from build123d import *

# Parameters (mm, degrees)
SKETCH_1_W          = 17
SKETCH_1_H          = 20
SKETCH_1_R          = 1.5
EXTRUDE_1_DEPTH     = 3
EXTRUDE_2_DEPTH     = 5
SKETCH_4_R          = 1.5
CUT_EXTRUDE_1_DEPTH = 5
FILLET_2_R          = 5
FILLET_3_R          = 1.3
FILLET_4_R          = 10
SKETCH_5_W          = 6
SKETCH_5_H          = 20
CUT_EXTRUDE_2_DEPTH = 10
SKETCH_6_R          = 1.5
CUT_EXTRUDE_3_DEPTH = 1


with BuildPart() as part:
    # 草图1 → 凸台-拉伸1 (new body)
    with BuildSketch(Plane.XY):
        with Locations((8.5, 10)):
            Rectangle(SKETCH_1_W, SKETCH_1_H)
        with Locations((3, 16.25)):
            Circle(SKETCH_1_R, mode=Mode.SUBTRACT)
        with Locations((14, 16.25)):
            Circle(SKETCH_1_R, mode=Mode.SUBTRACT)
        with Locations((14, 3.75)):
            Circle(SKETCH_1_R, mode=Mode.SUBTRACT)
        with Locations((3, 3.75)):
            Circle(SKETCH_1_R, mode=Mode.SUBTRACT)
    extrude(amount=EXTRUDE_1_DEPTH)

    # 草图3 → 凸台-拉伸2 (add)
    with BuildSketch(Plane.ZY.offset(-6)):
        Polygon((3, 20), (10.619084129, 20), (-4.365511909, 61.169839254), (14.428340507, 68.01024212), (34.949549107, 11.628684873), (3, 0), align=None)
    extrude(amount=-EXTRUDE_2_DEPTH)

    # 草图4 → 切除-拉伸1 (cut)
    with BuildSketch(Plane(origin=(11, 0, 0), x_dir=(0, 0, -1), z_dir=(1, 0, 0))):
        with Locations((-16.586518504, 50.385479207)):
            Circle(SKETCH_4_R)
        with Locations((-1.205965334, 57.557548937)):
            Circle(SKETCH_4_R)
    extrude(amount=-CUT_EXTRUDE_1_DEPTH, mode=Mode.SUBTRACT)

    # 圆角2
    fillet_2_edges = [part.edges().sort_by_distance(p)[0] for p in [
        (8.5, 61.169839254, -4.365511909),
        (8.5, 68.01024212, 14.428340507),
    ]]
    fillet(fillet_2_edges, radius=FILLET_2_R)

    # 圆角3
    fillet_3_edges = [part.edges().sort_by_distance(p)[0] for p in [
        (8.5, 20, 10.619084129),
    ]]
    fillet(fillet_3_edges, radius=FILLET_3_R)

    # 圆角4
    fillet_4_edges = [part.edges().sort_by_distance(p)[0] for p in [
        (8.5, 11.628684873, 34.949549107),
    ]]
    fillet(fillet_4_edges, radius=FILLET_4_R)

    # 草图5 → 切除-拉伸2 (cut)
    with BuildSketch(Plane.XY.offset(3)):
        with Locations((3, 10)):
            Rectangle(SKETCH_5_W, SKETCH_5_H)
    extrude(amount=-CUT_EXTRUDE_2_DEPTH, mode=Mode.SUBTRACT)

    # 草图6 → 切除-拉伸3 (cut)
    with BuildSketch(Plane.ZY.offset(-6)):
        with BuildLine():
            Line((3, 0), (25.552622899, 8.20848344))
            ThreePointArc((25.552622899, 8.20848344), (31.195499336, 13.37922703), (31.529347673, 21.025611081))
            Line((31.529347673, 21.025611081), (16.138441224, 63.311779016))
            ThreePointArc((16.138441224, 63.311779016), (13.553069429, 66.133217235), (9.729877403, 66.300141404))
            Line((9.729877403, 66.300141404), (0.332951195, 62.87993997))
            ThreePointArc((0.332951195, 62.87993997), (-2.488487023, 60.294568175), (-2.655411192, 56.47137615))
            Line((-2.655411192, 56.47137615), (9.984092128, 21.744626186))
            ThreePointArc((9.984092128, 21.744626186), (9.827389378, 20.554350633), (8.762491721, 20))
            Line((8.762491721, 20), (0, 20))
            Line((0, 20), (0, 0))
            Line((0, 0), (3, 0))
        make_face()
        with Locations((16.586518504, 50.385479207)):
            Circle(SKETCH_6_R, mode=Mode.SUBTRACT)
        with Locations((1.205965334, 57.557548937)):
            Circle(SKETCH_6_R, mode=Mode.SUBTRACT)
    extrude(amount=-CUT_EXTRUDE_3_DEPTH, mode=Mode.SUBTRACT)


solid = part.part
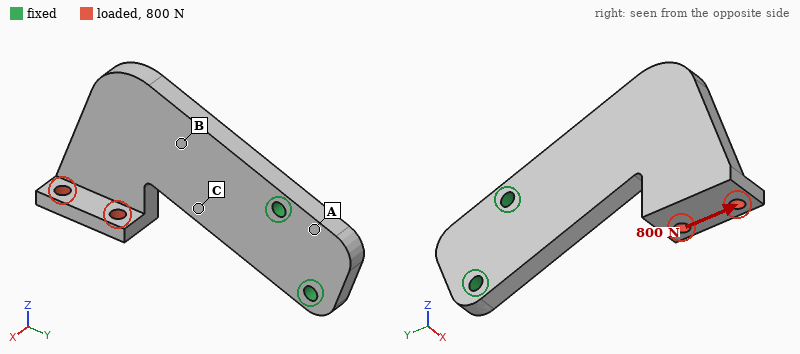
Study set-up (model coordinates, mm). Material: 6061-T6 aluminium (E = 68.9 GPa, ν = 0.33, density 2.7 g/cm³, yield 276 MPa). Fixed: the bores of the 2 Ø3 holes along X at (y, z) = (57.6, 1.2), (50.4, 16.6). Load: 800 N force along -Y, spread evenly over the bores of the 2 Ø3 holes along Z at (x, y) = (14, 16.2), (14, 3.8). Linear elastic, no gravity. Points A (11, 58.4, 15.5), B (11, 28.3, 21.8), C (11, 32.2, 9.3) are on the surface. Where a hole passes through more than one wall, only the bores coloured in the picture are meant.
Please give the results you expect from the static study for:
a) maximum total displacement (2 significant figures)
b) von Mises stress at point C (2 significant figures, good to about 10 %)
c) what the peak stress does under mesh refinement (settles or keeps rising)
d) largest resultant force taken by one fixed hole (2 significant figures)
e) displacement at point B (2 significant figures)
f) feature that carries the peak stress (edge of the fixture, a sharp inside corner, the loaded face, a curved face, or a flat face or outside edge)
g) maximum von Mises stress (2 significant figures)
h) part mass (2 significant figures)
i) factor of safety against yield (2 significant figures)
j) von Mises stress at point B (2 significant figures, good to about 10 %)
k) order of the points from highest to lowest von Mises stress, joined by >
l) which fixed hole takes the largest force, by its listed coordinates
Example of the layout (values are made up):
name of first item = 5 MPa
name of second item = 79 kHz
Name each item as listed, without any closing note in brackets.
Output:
maximum total displacement = 0.80 mm
von Mises stress at point C = 120 MPa
what the peak stress does under mesh refinement = settles
largest resultant force taken by one fixed hole = 790 N
displacement at point B = 0.14 mm
feature that carries the peak stress = a curved face
maximum von Mises stress = 430 MPa
part mass = 16 g
factor of safety against yield = 0.64
von Mises stress at point B = 60 MPa
order of the points from highest to lowest von Mises stress, joined by > = C > B > A
which fixed hole takes the largest force, by its listed coordinates = (57.6, 1.2)
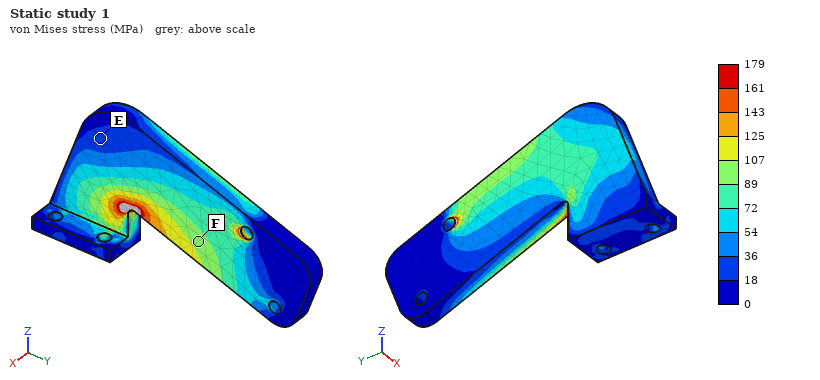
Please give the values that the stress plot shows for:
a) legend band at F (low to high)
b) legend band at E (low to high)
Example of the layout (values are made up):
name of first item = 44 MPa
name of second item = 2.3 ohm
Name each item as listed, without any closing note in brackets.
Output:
legend band at F = 89 to 107 MPa
legend band at E = 18 to 36 MPa
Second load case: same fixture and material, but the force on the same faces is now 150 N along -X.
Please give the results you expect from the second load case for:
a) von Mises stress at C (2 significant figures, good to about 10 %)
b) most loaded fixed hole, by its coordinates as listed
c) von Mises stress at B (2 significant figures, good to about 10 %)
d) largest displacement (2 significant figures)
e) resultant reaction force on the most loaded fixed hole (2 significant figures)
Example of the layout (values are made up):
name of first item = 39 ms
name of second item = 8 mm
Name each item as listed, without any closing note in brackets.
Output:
von Mises stress at C = 77 MPa
most loaded fixed hole, by its coordinates as listed = (50.4, 16.6)
von Mises stress at B = 54 MPa
largest displacement = 0.82 mm
resultant reaction force on the most loaded fixed hole = 200 N
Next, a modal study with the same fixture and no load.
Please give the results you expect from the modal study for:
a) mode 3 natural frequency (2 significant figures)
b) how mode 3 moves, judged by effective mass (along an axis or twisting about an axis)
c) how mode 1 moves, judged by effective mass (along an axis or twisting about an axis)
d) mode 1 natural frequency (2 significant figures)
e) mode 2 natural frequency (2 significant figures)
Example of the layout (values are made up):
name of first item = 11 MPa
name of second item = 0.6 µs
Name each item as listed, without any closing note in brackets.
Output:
mode 3 natural frequency = 4500 Hz
how mode 3 moves, judged by effective mass = along Z
how mode 1 moves, judged by effective mass = along X
mode 1 natural frequency = 1100 Hz
mode 2 natural frequency = 3300 Hz
